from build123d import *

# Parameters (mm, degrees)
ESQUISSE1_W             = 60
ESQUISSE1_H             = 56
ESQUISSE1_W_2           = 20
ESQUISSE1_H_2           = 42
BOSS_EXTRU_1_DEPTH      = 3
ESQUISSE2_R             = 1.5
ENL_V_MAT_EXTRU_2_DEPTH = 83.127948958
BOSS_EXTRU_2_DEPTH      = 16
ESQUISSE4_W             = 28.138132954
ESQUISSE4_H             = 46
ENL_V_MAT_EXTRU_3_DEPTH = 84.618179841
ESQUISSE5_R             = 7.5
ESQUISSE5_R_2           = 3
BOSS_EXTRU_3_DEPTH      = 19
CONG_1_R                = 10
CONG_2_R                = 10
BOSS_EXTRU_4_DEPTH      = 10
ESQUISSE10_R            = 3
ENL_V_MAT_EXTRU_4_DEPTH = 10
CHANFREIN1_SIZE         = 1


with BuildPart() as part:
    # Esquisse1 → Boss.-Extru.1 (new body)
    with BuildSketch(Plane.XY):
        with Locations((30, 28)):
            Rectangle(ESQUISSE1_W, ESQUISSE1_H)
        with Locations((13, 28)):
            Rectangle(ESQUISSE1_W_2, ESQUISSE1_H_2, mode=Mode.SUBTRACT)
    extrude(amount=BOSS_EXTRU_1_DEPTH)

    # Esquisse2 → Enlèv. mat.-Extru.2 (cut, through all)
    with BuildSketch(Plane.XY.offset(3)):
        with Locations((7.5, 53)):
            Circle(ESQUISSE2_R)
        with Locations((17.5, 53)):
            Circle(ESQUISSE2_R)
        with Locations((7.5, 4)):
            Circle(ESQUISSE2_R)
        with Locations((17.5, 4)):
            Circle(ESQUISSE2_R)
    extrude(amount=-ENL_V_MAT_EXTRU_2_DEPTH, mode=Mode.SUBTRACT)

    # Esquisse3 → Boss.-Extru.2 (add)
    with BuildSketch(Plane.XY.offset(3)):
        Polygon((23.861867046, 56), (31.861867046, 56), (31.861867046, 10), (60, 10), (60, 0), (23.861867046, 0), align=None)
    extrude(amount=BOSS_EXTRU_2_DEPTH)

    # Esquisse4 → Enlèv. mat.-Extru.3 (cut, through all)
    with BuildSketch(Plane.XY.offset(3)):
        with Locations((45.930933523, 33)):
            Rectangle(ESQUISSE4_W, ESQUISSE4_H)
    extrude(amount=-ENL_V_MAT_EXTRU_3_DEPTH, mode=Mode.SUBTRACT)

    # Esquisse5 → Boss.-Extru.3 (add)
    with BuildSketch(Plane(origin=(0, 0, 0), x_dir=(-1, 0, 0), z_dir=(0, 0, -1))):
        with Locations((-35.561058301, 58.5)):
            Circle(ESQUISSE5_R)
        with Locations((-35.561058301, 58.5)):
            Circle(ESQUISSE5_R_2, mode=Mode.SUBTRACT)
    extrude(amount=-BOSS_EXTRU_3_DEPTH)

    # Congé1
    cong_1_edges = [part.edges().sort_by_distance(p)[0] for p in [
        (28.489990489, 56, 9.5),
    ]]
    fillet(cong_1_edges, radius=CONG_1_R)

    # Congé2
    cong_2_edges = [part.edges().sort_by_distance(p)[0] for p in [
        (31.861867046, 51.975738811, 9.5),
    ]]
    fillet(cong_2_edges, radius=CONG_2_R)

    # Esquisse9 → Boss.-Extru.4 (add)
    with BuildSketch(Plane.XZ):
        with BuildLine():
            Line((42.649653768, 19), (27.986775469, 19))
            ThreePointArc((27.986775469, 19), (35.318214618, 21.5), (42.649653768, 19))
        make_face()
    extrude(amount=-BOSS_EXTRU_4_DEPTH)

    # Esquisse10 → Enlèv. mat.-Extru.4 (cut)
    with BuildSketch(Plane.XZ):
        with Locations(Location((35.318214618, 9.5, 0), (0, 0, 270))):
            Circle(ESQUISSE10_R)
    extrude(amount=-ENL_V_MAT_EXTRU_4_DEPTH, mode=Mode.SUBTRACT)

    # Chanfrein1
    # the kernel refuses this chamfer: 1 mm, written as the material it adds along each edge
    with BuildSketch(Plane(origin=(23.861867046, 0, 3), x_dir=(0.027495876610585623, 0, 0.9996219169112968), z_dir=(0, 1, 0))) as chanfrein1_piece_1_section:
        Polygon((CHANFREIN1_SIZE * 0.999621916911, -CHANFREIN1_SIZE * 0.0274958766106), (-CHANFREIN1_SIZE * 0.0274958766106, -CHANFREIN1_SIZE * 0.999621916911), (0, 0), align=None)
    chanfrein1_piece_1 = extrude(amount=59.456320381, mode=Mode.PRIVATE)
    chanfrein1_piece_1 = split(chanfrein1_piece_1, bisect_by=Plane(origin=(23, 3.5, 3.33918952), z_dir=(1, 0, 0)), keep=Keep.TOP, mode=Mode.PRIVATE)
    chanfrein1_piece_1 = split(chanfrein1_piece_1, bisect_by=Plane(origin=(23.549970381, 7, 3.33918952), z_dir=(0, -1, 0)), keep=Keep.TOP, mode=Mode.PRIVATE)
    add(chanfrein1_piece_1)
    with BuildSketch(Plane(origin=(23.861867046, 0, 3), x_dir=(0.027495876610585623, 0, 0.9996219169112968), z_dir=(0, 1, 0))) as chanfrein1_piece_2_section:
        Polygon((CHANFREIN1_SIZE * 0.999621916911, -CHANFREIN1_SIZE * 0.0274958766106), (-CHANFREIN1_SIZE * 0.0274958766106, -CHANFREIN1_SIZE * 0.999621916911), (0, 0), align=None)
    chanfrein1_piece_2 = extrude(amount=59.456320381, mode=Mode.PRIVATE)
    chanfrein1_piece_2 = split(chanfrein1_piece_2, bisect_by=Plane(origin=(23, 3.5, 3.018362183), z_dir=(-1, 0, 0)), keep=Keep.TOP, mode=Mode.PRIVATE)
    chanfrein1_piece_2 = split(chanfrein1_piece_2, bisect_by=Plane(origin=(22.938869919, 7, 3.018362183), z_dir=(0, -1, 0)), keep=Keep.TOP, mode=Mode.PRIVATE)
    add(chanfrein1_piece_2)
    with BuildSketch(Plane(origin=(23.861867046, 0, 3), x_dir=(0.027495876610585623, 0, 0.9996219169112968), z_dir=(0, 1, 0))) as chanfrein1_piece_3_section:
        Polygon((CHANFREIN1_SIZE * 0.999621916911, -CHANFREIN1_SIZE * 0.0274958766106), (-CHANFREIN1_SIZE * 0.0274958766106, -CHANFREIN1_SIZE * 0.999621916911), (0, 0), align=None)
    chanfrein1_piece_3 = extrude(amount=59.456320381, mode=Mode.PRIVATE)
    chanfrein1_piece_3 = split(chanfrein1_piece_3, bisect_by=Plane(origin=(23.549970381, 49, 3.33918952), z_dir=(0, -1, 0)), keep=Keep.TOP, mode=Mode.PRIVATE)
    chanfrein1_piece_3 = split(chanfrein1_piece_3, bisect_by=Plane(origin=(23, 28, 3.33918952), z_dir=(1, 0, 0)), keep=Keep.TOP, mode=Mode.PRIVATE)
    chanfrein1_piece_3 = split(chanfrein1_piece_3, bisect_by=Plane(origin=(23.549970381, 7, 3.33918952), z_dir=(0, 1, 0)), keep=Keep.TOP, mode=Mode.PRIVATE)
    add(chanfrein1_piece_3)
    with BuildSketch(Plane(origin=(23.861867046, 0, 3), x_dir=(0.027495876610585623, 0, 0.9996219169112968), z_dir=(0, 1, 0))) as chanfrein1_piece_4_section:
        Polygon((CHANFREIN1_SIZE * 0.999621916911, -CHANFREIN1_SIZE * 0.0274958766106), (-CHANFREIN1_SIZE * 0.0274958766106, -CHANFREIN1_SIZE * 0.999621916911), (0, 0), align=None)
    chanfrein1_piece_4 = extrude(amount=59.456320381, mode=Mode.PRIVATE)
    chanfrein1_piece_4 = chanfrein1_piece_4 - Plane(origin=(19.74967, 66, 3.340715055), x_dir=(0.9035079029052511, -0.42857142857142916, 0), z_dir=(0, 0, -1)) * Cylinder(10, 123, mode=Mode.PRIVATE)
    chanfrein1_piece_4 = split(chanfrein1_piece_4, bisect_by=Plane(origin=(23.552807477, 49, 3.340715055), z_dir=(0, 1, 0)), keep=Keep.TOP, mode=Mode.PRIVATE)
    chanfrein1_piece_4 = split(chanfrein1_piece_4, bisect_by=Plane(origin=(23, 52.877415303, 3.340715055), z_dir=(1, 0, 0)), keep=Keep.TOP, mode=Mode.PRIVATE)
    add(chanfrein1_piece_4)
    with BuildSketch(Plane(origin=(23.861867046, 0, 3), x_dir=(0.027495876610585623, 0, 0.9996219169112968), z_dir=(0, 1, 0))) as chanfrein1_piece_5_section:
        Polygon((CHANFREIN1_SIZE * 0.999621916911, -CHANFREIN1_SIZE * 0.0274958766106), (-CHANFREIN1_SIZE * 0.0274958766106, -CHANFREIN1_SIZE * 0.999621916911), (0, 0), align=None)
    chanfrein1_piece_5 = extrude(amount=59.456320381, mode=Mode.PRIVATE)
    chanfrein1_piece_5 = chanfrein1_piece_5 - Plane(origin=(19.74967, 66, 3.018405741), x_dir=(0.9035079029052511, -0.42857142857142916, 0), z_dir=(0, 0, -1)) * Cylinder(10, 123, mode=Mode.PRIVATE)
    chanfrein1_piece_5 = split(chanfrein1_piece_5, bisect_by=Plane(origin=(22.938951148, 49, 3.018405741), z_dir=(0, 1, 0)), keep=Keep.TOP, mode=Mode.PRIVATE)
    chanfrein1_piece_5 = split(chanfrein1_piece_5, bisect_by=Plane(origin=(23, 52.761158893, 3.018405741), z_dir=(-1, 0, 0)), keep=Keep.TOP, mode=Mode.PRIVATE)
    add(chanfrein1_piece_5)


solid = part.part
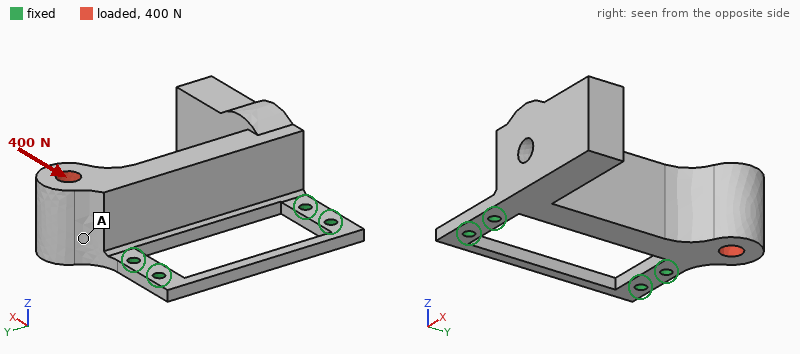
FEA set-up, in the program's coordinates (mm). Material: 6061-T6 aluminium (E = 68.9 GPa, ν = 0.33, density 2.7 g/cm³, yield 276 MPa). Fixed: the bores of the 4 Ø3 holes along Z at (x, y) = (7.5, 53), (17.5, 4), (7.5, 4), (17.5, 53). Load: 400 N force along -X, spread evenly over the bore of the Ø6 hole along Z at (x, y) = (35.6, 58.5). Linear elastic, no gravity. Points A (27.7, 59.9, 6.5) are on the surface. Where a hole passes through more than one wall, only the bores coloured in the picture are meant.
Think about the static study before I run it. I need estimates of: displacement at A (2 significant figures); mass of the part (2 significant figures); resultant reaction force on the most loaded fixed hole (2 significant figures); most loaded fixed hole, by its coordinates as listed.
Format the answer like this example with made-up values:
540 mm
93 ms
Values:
0.080 mm
50 g
430 N
(17.5, 53)
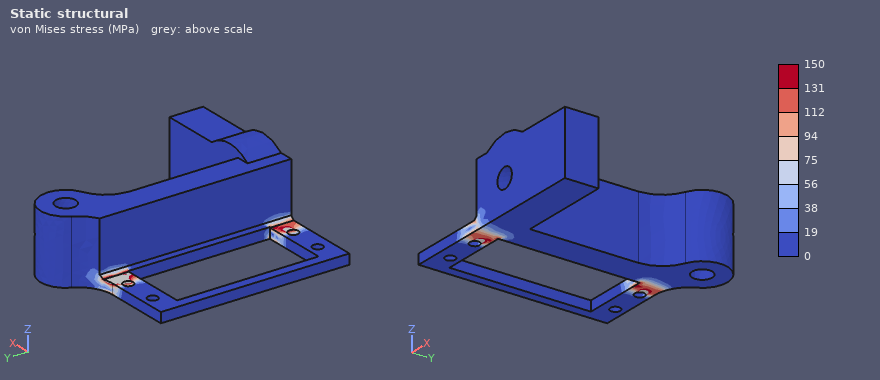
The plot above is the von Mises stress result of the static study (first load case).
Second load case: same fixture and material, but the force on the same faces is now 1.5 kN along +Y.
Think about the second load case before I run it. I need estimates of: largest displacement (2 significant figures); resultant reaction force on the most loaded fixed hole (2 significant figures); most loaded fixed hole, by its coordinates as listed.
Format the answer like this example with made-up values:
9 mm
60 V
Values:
72 µm
1.1 kN
(17.5, 4)
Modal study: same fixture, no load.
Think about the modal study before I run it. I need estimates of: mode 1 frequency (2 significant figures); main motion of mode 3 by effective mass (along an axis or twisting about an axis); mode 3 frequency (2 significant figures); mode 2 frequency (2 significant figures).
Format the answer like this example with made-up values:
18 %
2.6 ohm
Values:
730 Hz
along Y
3800 Hz
3400 Hz
